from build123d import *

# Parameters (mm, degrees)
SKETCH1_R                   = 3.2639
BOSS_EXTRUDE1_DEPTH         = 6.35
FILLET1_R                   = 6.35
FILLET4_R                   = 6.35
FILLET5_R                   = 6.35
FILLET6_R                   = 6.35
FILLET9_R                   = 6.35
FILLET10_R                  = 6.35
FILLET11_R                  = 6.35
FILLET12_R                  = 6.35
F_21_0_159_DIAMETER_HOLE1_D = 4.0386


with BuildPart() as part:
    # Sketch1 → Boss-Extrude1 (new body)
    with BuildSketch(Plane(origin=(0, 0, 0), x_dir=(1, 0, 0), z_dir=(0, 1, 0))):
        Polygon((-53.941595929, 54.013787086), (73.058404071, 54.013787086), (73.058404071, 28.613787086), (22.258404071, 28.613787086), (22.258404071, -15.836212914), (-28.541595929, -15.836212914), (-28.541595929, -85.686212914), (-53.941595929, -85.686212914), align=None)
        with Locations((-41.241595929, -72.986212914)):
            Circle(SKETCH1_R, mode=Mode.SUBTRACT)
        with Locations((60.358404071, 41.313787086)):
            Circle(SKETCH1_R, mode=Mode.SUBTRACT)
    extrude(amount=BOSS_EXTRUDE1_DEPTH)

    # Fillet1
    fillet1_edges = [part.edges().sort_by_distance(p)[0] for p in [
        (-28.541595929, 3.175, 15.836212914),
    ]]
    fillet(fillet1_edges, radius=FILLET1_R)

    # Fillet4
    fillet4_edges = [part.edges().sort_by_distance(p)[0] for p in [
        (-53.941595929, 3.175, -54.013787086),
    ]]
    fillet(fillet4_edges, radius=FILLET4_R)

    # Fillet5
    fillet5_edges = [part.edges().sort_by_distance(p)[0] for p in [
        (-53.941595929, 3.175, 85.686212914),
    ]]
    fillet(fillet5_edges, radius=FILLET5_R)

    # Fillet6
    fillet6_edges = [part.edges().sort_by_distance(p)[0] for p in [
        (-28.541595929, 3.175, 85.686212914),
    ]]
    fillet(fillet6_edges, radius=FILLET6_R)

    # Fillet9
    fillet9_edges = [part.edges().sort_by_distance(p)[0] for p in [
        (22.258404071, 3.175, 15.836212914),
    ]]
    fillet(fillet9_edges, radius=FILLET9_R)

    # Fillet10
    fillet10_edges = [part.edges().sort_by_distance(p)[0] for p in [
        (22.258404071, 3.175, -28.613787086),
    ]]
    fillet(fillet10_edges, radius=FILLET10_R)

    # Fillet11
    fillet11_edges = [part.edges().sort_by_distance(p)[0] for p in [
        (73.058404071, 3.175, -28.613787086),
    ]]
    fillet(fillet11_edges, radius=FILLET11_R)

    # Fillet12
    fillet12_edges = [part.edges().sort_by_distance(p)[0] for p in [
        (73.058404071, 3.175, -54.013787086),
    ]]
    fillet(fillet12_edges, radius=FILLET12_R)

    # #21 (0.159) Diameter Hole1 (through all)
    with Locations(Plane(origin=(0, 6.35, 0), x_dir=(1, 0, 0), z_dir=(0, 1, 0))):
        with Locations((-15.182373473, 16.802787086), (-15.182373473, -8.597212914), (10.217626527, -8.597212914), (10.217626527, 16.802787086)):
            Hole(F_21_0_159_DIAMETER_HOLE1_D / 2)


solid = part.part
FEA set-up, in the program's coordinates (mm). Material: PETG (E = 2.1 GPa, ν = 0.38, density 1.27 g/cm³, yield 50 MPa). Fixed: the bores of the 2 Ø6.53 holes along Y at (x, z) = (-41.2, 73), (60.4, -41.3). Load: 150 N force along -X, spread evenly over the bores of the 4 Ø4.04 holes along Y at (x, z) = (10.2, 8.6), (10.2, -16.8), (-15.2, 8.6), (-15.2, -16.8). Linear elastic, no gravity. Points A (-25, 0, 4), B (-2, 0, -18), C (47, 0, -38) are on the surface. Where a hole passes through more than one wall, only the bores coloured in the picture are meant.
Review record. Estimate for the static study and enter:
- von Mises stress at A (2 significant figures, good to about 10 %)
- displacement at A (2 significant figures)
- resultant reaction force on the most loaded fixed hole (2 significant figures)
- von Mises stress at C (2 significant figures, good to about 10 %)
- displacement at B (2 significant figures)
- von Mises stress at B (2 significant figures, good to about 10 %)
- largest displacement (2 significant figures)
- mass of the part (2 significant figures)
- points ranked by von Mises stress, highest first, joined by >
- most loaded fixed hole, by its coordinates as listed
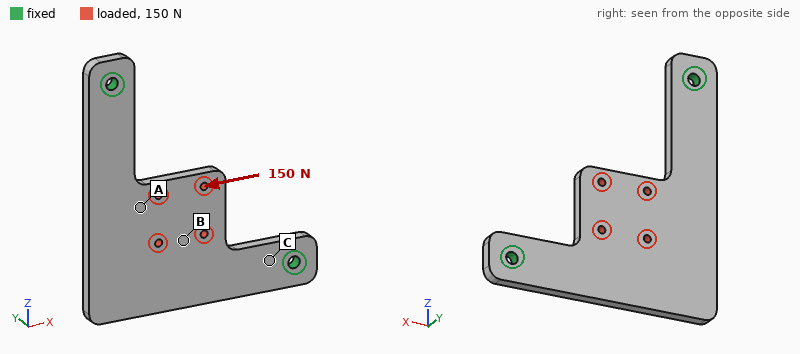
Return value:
0.25 MPa
54 µm
130 N
1.2 MPa
39 µm
0.46 MPa
70 µm
66 g
C > B > A
(60.4, -41.3)
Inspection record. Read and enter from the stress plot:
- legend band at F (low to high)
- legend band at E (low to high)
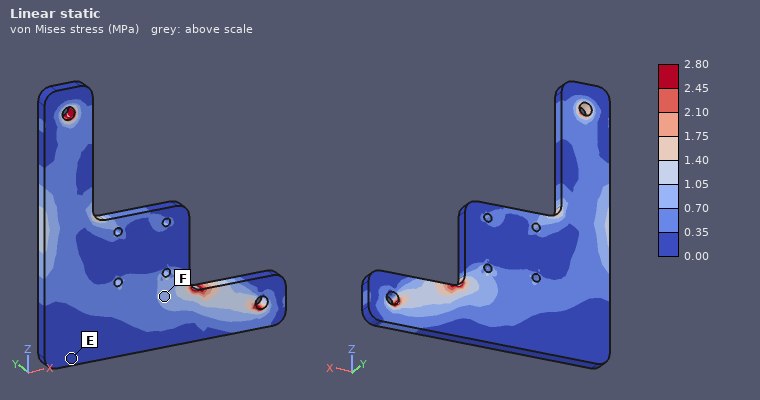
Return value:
0.70 to 1.05 MPa
0.00 to 0.35 MPa
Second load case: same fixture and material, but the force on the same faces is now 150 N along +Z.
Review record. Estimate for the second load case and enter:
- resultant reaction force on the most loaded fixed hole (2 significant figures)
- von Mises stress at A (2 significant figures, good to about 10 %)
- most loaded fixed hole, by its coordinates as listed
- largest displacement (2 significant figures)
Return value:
110 N
0.69 MPa
(-41.2, 73)
65 µm
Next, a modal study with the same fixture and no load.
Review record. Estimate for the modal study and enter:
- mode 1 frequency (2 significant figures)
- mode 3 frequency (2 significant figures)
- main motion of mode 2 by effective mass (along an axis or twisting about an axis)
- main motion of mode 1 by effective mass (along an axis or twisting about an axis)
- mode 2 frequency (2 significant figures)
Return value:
140 Hz
560 Hz
along Y
along Y
370 Hz
